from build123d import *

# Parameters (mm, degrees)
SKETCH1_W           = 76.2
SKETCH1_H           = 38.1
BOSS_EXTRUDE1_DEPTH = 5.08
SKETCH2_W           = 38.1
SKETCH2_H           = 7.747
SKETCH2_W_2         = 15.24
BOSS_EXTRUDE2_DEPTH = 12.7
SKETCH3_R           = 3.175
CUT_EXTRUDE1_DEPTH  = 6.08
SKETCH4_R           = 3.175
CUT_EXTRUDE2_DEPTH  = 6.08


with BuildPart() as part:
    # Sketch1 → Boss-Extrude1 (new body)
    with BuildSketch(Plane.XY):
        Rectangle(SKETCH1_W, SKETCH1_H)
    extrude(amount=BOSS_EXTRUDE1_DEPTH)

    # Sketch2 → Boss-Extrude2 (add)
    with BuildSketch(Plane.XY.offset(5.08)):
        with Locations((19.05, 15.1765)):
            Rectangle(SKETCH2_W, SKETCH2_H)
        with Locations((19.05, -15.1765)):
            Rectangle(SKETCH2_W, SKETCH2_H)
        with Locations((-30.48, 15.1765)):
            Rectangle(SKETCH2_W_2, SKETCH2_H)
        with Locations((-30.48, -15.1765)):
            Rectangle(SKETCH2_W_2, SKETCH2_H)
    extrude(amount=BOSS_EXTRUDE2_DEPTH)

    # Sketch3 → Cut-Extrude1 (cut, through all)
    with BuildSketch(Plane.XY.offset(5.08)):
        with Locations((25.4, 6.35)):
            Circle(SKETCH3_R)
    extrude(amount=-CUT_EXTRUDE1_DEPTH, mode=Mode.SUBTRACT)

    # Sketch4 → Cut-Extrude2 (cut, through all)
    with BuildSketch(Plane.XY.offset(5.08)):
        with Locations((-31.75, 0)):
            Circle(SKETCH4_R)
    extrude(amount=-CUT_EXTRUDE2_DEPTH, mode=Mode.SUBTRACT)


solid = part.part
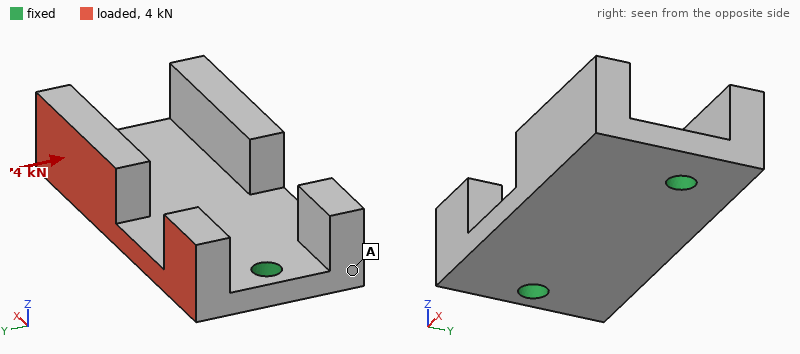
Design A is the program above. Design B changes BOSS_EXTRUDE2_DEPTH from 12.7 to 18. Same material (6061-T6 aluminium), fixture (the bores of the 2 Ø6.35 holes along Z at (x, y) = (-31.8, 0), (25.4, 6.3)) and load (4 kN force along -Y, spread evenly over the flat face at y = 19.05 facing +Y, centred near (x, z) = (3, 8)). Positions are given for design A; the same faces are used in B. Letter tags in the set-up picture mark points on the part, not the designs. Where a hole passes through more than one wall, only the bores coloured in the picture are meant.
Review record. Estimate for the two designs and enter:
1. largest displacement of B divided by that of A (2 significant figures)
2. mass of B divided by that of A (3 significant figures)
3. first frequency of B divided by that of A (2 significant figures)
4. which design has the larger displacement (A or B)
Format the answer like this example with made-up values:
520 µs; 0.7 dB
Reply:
1.8; 1.18; 0.81; B
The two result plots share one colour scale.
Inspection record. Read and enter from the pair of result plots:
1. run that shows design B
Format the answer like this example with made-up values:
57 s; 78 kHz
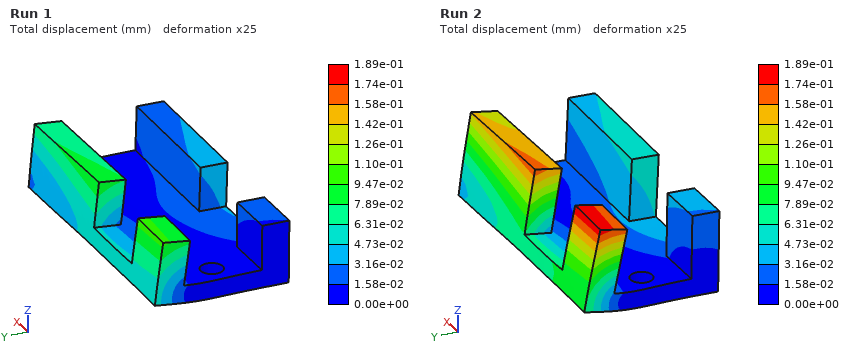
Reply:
Run 2
